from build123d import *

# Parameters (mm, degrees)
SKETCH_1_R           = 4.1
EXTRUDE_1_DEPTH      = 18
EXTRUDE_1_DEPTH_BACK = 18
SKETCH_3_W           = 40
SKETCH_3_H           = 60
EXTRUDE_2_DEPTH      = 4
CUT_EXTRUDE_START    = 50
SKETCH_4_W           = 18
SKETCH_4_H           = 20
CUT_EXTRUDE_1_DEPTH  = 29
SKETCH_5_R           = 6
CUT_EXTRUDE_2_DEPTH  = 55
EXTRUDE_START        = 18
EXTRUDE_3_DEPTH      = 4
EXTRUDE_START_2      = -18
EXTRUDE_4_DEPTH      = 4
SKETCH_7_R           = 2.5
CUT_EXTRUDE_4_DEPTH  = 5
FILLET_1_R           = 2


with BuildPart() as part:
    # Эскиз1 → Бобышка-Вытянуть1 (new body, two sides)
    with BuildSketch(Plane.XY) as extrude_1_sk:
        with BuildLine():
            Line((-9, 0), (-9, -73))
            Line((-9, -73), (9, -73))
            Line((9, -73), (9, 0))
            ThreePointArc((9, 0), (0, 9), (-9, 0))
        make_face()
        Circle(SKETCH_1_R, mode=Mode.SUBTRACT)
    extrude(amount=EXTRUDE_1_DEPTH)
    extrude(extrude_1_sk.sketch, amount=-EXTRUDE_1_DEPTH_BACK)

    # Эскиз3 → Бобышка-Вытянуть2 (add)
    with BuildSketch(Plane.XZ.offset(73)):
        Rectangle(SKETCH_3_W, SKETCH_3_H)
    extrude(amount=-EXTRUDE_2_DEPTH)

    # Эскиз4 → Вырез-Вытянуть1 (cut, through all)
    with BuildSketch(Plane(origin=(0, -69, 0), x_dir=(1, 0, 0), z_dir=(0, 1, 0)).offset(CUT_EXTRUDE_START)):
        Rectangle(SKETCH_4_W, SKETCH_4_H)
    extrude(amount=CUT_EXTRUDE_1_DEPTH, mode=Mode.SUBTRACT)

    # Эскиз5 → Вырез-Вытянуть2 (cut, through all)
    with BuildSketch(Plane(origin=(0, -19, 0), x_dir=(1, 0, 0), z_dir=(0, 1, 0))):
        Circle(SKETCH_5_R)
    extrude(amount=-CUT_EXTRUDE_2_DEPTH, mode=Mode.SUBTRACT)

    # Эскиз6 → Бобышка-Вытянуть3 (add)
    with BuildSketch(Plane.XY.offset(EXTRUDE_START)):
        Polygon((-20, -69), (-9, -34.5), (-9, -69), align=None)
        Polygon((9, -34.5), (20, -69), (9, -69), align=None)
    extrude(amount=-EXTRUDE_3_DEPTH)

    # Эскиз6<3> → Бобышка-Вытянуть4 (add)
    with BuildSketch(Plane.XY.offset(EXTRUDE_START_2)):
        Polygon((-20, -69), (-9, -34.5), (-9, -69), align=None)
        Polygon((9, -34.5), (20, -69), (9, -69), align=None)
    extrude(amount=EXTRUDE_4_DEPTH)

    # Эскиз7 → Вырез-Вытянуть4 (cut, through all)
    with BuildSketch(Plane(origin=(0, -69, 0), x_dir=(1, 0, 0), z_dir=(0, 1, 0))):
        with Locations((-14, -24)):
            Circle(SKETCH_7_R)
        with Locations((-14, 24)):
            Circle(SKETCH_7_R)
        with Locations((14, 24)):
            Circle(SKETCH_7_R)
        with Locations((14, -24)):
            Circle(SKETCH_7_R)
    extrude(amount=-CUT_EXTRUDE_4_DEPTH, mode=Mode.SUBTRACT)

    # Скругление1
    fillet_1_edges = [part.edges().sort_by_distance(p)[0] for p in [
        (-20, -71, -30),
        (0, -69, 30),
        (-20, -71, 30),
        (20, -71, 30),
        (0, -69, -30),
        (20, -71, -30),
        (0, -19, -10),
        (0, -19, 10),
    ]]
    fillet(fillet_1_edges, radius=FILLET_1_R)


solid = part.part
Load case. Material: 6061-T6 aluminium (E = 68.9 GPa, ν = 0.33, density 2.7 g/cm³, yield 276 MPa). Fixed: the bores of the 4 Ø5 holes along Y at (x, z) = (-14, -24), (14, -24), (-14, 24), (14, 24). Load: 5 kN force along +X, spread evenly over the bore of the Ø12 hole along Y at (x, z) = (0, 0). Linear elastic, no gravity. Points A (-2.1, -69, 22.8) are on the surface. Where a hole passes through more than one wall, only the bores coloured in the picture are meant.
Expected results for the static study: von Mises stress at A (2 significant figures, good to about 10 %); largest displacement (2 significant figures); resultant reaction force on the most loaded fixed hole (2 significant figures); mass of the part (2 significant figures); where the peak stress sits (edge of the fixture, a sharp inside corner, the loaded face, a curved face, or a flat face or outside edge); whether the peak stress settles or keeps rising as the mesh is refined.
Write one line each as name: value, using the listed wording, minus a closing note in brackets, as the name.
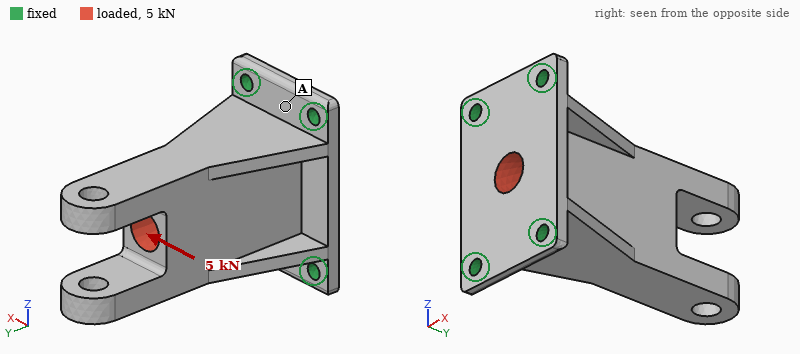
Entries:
von Mises stress at A: 39 MPa
largest displacement: 0.22 mm
resultant reaction force on the most loaded fixed hole: 2.7 kN
mass of the part: 120 g
where the peak stress sits: edge of the fixture
whether the peak stress settles or keeps rising as the mesh is refined: keeps rising
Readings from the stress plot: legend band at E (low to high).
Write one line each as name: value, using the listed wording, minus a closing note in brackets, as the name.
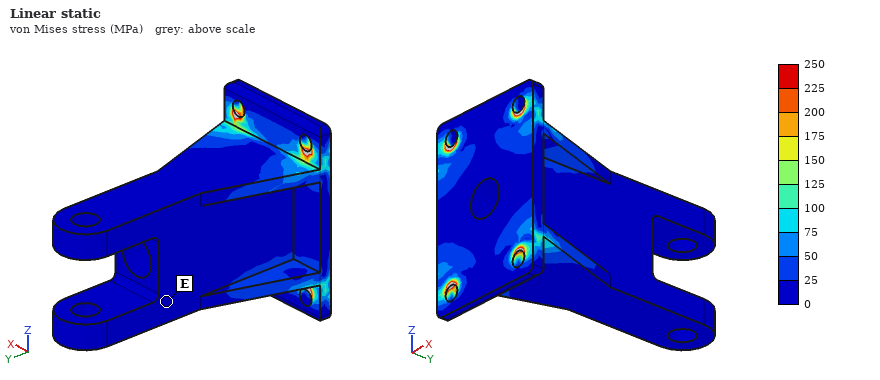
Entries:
legend band at E: 0 to 25 MPa
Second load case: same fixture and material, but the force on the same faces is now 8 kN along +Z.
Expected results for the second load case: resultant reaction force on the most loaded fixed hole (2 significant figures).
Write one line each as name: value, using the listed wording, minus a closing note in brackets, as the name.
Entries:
resultant reaction force on the most loaded fixed hole: 3.3 kN
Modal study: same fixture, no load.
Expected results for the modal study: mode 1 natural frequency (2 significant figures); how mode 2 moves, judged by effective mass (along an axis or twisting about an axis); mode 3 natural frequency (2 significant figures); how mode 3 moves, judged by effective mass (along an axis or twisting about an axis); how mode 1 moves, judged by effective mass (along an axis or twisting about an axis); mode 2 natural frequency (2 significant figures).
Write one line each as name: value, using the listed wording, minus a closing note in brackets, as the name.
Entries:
mode 1 natural frequency: 2600 Hz
how mode 2 moves, judged by effective mass: along Z
mode 3 natural frequency: 6500 Hz
how mode 3 moves, judged by effective mass: twisting about Y
how mode 1 moves, judged by effective mass: along X
mode 2 natural frequency: 3500 Hz
